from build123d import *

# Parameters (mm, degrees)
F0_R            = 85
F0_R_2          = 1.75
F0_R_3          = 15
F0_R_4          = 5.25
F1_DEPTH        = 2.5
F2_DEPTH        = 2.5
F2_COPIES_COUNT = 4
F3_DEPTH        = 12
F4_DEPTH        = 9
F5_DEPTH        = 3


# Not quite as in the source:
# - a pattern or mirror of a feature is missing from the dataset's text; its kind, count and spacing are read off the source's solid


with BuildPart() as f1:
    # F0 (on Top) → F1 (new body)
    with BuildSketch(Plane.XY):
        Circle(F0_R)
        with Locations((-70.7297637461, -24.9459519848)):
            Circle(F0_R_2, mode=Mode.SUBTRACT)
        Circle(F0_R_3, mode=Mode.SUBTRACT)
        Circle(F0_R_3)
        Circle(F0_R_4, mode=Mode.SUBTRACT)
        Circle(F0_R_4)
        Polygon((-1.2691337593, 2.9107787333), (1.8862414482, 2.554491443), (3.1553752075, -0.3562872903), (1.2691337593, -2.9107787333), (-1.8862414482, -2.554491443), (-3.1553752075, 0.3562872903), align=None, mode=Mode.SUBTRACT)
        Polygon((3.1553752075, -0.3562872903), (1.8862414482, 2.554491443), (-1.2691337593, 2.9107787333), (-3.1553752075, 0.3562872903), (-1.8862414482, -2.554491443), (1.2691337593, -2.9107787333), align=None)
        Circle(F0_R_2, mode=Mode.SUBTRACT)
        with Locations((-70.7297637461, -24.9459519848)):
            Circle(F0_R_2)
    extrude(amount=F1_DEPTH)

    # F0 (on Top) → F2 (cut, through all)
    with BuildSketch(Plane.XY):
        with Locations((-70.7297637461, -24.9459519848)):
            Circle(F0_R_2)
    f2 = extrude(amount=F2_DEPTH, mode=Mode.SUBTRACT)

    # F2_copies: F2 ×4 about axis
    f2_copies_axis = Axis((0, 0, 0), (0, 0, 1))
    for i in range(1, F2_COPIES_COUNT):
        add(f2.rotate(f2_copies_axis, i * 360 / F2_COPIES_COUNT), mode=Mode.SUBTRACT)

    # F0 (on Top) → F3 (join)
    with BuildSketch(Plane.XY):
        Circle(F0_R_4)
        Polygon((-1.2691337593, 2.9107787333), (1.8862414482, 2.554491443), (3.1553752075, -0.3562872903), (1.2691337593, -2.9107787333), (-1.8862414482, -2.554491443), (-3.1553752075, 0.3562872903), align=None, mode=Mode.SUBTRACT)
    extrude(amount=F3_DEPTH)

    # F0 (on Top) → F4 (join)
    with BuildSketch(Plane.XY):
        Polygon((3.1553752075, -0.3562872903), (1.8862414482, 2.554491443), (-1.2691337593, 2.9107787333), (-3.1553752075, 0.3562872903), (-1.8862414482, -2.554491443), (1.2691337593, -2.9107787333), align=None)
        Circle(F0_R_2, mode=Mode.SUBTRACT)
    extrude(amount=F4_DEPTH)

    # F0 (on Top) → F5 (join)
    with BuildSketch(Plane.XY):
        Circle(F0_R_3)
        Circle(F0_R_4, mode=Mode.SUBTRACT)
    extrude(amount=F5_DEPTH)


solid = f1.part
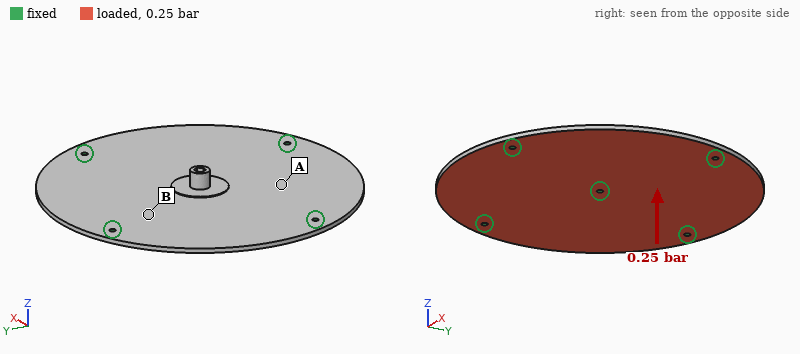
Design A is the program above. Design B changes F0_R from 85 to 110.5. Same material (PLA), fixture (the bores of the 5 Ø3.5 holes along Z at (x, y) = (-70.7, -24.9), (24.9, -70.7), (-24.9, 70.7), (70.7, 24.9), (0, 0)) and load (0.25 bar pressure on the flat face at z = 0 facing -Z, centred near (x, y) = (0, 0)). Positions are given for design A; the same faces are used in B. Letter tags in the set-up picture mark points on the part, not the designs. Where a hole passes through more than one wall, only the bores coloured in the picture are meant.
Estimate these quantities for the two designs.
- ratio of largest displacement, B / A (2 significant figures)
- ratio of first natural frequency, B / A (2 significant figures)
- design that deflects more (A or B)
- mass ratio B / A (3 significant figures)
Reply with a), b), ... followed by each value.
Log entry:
a) 2.8
b) 0.55
c) B
d) 1.68
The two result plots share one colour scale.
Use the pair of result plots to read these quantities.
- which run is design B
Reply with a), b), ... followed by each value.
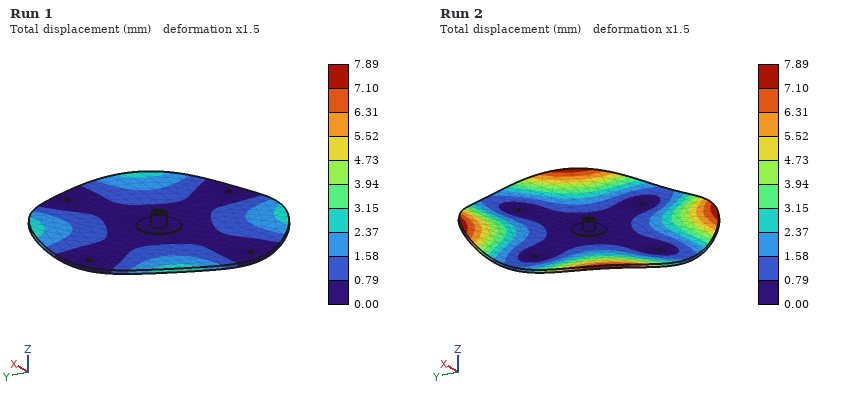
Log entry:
a) Run 2
